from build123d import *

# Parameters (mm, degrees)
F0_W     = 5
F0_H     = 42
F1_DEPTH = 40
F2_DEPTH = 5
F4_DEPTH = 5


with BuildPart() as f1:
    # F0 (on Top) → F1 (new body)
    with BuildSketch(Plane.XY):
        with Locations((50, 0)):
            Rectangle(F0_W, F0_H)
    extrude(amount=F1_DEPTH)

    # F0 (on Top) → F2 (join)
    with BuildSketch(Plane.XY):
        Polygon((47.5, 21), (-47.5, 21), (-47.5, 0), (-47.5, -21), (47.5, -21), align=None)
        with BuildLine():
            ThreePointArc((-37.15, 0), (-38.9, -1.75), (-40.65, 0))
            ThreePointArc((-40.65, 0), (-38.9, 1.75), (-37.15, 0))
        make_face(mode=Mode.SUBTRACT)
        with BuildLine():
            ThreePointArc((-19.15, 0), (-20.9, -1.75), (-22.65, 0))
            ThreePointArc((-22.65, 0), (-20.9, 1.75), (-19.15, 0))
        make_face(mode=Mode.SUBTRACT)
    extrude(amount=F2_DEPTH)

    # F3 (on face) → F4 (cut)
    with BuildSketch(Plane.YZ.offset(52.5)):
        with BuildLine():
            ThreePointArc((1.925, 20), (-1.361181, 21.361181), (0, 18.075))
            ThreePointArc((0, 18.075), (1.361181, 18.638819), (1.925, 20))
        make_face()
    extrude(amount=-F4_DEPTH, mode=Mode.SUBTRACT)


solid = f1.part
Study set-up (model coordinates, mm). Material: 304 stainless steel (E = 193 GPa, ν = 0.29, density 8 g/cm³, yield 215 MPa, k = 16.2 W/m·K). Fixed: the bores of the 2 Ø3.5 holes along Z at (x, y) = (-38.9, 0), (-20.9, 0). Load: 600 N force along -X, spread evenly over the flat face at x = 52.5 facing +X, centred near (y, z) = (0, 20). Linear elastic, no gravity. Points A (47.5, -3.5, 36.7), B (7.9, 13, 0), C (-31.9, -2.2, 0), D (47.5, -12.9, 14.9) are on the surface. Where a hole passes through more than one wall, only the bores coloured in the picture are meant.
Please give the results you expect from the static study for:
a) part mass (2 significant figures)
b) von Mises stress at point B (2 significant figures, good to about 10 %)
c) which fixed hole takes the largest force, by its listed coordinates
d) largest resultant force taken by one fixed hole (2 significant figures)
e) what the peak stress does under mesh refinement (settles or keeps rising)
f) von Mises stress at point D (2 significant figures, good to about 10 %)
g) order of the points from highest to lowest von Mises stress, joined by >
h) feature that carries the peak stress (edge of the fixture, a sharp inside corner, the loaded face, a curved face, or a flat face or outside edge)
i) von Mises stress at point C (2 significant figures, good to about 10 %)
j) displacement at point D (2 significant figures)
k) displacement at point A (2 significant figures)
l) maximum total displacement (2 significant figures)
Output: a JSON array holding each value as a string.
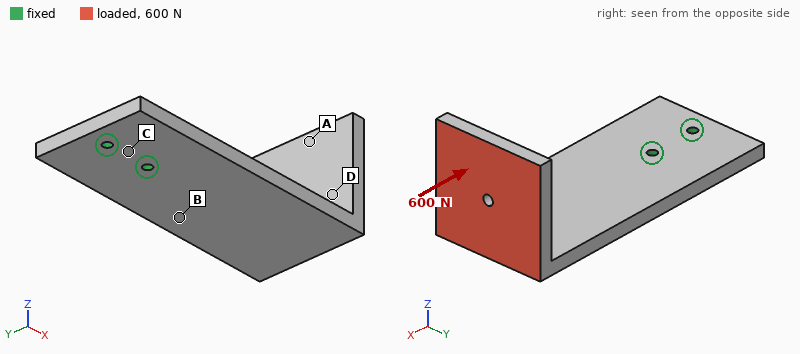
["230 g", "56 MPa", "(-20.9, 0)", "530 N", "keeps rising", "26 MPa", "B > D > C > A", "edge of the fixture", "16 MPa", "0.33 mm", "0.45 mm", "0.51 mm"]
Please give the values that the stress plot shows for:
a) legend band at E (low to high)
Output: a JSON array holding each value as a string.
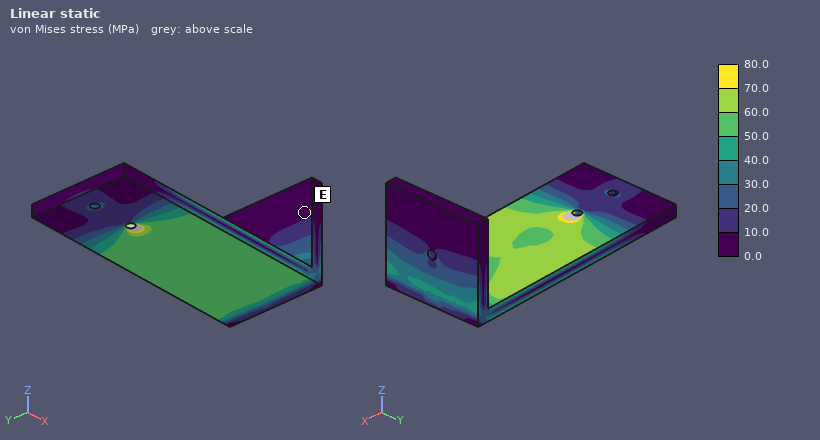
["0.0 to 10.0 MPa"]
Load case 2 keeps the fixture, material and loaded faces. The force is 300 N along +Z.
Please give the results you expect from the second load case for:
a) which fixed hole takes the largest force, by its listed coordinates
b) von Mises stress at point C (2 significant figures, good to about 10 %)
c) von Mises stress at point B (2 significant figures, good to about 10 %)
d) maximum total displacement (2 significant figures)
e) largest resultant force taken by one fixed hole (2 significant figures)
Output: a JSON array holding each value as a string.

["(-20.9, 0)", "28 MPa", "75 MPa", "0.64 mm", "930 N"]
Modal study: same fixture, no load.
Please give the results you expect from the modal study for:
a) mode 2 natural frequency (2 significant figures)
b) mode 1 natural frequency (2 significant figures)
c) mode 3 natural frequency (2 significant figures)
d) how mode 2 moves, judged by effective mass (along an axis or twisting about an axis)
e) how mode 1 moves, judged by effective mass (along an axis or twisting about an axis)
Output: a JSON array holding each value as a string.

["940 Hz", "400 Hz", "1600 Hz", "along Y", "along Z"]
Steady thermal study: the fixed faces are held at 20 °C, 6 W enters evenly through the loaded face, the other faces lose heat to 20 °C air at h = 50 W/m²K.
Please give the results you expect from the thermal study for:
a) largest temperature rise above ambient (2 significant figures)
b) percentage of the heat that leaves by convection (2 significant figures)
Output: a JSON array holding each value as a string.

["33 K", "95 %"]
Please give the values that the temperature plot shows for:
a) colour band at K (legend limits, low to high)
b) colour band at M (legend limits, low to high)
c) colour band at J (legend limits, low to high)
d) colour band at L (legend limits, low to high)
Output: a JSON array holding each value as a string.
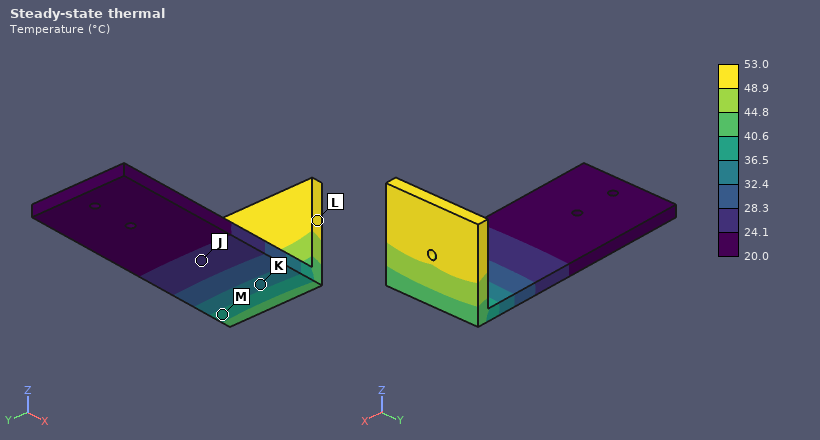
["32.4 to 36.5 °C", "36.5 to 40.6 °C", "24.1 to 28.3 °C", "48.9 to 53.0 °C"]
